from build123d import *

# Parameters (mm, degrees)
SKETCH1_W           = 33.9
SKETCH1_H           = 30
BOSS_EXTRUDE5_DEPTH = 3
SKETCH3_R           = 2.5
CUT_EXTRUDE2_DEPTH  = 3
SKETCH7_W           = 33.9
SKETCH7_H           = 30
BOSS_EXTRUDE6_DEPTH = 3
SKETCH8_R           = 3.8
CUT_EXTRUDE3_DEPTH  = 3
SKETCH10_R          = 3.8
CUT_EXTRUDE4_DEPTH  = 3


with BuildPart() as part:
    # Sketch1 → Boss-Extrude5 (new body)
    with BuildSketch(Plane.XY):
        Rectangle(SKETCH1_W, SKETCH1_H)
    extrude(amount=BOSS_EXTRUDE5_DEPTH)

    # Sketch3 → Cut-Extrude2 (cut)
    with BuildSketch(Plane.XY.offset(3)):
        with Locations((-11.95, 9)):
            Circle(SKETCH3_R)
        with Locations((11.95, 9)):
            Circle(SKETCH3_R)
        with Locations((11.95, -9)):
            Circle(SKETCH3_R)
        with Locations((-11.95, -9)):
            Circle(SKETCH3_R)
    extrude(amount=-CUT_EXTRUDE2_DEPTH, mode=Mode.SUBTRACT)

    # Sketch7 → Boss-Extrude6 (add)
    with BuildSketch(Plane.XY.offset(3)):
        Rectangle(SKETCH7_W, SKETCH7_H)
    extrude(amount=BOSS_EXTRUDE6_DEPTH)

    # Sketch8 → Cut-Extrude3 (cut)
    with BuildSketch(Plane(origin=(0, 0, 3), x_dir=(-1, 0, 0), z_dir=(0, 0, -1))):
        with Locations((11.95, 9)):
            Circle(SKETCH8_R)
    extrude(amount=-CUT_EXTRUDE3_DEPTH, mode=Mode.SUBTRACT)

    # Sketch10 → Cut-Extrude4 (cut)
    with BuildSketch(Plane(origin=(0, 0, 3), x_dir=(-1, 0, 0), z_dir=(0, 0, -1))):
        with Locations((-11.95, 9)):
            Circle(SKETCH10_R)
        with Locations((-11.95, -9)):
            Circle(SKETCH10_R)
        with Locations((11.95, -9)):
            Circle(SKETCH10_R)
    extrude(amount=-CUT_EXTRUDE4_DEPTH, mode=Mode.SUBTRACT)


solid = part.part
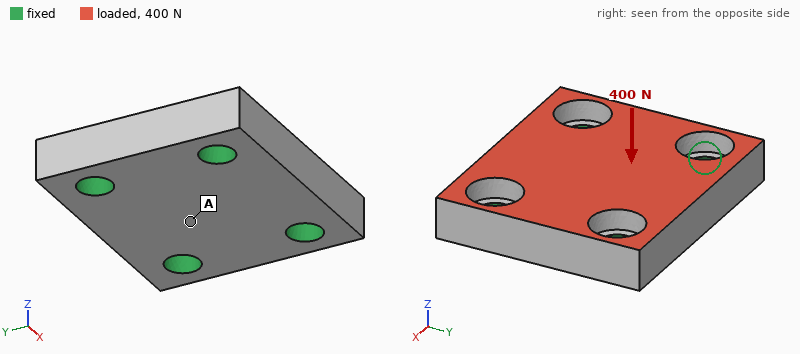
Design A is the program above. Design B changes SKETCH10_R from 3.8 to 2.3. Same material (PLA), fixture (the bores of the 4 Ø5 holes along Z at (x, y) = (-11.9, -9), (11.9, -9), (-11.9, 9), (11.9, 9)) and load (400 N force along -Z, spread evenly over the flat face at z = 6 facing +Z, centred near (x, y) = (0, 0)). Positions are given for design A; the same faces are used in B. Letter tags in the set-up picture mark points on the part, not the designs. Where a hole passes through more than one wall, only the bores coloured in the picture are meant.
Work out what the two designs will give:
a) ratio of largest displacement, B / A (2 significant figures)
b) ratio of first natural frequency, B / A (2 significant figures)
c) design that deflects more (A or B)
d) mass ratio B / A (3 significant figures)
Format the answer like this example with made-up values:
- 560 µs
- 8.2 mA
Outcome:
- 0.84
- 1.1
- A
- 1.05
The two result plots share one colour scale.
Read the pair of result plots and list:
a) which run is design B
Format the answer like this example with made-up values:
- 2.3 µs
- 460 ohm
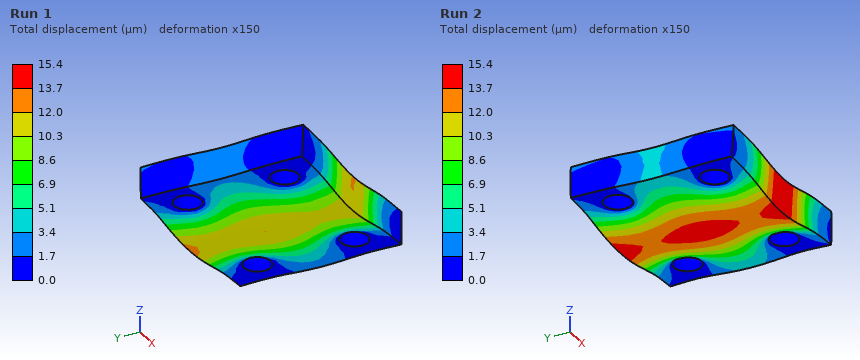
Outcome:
- Run 1
